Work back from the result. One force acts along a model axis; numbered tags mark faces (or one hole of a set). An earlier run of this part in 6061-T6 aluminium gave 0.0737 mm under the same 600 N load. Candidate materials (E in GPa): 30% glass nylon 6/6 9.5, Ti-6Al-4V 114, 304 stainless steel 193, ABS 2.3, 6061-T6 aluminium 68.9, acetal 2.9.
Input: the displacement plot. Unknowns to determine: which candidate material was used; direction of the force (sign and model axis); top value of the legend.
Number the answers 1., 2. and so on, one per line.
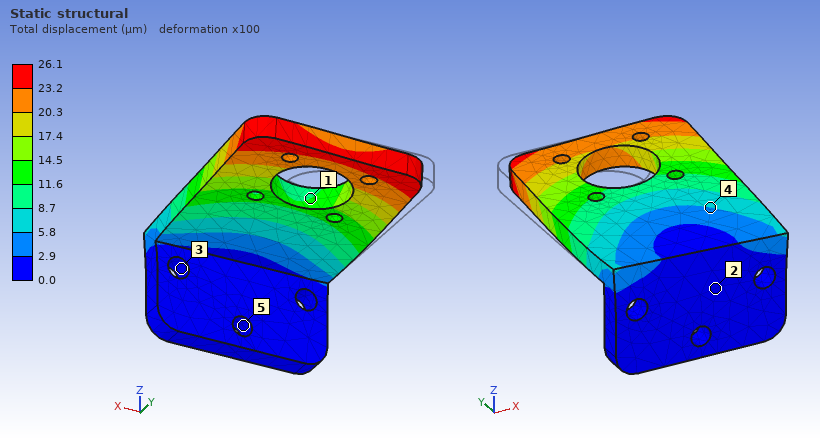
1. 304 stainless steel
2. +X
3. 26.1 µm
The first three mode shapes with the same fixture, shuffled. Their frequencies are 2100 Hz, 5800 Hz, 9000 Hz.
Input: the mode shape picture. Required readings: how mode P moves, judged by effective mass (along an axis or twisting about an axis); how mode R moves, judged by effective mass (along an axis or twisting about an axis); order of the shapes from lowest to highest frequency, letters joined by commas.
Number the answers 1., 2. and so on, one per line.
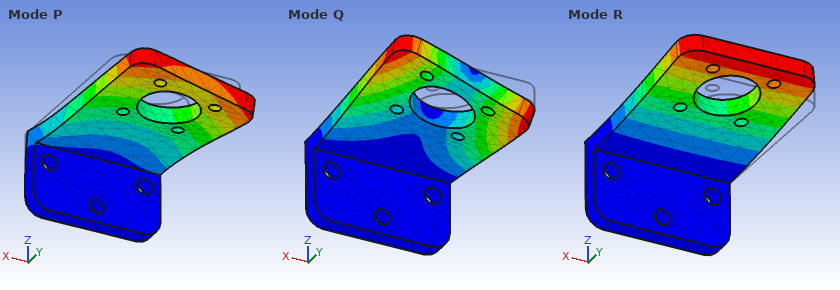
1. along X
2. along Z
3. R, Q, P
